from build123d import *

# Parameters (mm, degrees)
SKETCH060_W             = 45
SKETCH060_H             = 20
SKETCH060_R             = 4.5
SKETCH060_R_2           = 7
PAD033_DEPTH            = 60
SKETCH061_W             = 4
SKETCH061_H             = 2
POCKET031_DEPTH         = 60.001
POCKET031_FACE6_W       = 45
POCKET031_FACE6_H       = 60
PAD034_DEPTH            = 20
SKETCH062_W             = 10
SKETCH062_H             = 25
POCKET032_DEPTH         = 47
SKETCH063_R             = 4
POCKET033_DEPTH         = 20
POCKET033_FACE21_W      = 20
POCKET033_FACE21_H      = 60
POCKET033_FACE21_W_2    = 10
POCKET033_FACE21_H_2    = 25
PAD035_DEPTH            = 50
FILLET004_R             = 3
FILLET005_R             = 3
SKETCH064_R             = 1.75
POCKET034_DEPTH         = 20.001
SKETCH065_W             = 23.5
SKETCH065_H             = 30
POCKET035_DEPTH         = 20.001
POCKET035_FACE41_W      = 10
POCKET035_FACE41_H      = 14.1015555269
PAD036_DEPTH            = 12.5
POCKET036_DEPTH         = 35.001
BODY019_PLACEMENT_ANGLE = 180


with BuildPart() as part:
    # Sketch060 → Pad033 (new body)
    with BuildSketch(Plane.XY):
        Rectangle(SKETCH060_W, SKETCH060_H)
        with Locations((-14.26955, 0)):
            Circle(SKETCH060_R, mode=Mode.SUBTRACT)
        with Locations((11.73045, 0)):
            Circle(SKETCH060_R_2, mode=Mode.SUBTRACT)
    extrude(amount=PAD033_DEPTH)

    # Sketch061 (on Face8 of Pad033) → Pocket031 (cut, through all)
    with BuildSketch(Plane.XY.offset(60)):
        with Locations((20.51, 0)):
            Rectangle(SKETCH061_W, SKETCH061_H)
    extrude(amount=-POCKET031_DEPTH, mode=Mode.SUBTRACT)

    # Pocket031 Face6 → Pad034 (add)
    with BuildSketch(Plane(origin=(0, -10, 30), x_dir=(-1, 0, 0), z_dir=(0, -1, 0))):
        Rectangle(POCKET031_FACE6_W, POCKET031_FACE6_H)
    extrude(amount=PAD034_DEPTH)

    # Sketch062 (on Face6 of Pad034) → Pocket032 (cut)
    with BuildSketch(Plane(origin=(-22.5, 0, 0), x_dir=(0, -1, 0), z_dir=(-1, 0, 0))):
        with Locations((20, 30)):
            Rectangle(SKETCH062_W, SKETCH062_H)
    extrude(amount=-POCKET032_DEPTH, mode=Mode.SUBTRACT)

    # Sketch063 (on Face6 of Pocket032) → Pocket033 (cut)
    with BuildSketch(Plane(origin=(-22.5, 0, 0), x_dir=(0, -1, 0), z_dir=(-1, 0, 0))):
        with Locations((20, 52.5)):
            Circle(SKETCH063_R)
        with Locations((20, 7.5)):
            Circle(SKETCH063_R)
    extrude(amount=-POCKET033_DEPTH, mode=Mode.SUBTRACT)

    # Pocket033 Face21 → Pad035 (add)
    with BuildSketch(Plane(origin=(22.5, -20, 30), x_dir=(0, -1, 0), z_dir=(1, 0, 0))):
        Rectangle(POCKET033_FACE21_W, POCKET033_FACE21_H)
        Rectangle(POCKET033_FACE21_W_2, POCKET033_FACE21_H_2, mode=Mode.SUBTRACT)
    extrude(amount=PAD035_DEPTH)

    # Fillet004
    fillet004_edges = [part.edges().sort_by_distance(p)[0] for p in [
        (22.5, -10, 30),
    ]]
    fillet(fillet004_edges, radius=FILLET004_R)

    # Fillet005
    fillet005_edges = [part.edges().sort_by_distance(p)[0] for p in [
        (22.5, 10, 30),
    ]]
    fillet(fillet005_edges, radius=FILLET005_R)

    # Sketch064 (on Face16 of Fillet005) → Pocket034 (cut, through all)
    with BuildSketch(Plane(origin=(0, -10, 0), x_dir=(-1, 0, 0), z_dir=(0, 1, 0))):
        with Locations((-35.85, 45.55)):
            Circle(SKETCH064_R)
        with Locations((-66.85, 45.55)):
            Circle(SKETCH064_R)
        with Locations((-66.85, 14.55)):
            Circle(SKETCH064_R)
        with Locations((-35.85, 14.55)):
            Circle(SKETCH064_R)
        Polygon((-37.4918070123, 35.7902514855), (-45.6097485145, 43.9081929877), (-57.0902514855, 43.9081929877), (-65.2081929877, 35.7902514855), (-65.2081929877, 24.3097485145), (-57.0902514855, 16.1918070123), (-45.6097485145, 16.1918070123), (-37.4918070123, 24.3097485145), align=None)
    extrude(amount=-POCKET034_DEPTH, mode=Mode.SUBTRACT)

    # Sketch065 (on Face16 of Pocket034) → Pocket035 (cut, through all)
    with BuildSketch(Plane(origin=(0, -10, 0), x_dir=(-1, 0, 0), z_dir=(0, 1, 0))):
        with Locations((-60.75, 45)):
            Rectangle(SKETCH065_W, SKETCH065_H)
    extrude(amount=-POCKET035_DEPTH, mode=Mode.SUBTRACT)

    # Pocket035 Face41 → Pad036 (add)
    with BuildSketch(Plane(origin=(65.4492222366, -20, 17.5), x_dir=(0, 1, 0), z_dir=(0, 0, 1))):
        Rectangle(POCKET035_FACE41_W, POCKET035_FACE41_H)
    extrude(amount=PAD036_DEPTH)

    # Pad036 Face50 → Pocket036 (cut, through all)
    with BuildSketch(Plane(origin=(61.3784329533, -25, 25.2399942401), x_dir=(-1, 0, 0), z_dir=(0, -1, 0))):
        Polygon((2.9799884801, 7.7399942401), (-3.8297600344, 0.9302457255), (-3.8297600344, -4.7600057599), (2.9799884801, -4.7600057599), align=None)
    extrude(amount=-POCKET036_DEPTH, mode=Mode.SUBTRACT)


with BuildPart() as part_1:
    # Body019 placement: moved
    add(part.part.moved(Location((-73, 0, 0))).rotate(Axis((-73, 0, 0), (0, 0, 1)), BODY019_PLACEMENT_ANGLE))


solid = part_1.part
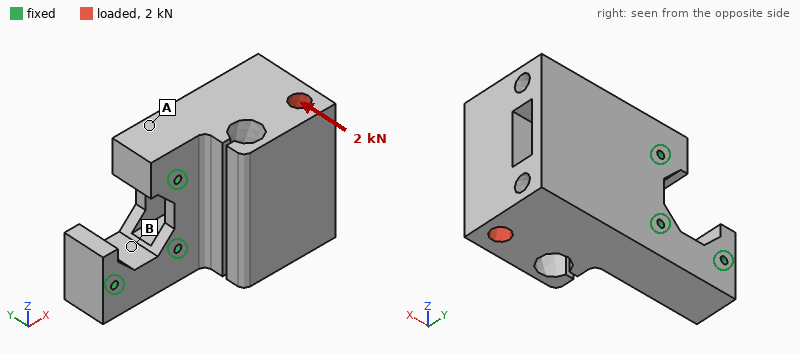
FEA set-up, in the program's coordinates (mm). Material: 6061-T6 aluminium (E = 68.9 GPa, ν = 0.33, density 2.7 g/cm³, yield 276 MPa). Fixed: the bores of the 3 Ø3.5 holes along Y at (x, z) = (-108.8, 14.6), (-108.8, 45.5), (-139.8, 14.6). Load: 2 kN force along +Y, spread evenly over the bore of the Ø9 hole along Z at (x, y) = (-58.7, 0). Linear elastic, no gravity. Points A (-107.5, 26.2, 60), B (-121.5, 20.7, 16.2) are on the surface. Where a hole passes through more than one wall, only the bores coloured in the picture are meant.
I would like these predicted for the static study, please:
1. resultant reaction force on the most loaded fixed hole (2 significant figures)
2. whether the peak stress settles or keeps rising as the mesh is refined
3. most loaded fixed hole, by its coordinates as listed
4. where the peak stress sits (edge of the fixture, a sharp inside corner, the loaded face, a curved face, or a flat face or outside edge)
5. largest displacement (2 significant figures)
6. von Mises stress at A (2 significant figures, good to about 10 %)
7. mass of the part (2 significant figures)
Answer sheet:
1.4 kN
keeps rising
(-108.8, 14.6)
edge of the fixture
68 µm
8.7 MPa
310 g
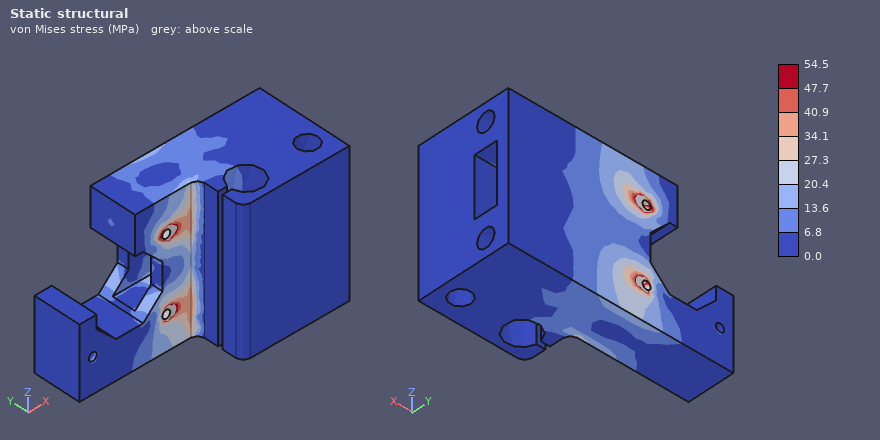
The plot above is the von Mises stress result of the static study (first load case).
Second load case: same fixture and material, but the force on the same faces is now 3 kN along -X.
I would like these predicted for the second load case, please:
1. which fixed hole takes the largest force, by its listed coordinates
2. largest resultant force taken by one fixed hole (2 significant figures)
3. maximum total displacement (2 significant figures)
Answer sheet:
(-108.8, 45.5)
1.6 kN
48 µm
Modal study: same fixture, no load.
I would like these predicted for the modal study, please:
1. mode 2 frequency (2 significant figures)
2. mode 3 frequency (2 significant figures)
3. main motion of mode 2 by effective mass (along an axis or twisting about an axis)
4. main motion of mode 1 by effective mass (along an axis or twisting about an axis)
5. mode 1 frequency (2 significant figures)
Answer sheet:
4800 Hz
6100 Hz
along Z
along Y
2700 Hz
